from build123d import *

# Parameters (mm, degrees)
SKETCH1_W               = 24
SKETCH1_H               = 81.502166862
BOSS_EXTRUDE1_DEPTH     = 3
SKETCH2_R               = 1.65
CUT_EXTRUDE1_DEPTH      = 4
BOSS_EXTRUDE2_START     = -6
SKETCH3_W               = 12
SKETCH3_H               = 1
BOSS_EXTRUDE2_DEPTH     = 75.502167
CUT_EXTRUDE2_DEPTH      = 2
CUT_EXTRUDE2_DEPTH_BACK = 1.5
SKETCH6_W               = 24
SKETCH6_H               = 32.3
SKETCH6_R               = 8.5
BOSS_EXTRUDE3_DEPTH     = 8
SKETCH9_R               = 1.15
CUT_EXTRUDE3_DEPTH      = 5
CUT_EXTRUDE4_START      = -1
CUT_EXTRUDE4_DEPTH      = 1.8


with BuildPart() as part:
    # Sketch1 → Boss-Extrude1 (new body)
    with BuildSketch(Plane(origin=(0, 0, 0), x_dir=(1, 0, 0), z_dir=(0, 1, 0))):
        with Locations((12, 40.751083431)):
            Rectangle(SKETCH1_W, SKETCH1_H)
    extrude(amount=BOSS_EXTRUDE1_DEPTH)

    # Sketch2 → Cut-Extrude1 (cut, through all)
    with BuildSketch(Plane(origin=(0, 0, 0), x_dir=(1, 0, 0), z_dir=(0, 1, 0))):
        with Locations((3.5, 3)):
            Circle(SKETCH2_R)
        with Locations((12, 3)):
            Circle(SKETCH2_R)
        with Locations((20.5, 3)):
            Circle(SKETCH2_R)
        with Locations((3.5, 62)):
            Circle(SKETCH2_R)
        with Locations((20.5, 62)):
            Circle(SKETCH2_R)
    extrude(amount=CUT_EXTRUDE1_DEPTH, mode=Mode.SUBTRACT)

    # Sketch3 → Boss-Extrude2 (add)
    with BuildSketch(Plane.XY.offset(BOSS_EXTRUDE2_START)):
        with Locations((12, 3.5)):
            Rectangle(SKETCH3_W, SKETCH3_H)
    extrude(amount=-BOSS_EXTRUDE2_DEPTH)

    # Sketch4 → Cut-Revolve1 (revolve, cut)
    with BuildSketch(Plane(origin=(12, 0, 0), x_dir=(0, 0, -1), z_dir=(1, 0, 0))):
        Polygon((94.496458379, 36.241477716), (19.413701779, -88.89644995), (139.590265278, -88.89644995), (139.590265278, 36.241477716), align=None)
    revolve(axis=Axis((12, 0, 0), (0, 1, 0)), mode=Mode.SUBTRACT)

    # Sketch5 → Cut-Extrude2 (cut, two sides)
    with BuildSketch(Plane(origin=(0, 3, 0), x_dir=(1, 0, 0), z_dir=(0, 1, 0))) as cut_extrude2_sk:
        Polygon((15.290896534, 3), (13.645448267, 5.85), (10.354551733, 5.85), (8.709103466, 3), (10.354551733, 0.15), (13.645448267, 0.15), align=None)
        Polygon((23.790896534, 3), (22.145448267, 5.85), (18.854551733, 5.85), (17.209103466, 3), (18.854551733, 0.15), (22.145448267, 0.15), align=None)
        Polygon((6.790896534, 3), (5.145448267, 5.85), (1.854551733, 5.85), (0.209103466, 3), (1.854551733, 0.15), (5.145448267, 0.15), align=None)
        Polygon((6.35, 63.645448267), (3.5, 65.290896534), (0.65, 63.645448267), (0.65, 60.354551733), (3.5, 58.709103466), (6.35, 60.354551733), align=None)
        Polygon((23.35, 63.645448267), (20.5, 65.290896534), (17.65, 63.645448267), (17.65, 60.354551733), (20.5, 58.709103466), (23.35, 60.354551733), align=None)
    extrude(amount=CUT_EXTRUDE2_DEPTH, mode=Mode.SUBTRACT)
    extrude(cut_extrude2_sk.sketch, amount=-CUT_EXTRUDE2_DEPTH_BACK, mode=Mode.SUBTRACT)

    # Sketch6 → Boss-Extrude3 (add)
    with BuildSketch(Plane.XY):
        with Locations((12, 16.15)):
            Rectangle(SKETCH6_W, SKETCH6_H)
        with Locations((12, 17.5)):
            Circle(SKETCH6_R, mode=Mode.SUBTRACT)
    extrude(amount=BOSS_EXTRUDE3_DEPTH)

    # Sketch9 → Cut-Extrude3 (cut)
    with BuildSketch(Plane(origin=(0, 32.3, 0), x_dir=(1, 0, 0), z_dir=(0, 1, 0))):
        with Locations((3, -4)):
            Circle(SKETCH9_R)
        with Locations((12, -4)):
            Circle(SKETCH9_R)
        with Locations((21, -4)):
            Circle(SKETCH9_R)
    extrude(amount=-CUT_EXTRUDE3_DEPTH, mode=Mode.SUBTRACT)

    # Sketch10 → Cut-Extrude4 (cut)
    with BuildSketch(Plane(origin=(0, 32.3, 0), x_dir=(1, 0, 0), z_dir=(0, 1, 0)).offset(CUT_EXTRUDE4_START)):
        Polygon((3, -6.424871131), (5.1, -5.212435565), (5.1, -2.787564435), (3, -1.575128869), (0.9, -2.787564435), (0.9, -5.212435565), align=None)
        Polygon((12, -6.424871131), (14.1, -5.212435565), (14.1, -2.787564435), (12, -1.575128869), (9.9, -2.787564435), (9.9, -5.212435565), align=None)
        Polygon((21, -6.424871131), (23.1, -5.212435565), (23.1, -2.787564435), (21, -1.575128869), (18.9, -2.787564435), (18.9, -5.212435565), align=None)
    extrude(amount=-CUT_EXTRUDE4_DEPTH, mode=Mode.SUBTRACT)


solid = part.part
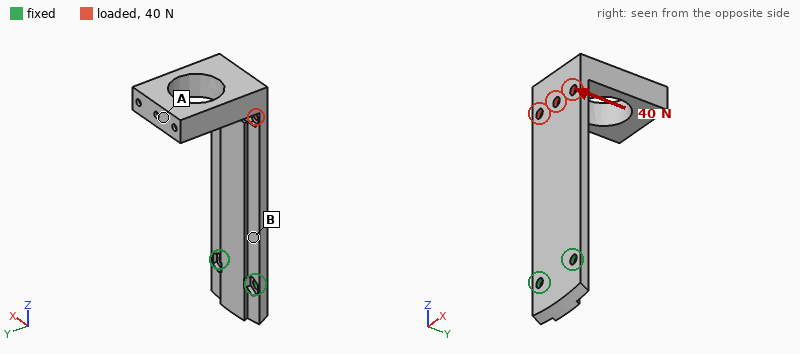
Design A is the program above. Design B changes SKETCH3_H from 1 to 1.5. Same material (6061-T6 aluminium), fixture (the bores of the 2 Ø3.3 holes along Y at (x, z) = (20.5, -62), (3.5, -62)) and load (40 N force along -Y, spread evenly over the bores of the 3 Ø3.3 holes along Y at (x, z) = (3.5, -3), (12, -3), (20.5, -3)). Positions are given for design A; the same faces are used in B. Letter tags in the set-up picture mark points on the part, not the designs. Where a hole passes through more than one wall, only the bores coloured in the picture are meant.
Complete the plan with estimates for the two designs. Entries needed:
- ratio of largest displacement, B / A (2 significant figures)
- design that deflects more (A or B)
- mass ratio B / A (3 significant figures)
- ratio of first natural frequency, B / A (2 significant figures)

0.90
A
1.02
1.1
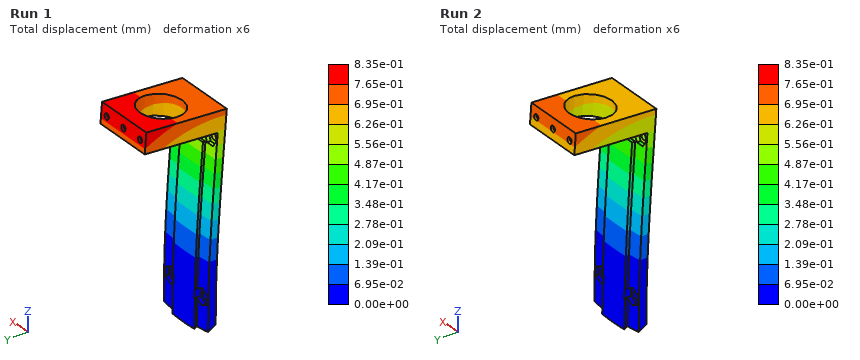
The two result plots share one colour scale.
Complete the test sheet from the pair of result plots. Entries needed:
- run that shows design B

Run 2
